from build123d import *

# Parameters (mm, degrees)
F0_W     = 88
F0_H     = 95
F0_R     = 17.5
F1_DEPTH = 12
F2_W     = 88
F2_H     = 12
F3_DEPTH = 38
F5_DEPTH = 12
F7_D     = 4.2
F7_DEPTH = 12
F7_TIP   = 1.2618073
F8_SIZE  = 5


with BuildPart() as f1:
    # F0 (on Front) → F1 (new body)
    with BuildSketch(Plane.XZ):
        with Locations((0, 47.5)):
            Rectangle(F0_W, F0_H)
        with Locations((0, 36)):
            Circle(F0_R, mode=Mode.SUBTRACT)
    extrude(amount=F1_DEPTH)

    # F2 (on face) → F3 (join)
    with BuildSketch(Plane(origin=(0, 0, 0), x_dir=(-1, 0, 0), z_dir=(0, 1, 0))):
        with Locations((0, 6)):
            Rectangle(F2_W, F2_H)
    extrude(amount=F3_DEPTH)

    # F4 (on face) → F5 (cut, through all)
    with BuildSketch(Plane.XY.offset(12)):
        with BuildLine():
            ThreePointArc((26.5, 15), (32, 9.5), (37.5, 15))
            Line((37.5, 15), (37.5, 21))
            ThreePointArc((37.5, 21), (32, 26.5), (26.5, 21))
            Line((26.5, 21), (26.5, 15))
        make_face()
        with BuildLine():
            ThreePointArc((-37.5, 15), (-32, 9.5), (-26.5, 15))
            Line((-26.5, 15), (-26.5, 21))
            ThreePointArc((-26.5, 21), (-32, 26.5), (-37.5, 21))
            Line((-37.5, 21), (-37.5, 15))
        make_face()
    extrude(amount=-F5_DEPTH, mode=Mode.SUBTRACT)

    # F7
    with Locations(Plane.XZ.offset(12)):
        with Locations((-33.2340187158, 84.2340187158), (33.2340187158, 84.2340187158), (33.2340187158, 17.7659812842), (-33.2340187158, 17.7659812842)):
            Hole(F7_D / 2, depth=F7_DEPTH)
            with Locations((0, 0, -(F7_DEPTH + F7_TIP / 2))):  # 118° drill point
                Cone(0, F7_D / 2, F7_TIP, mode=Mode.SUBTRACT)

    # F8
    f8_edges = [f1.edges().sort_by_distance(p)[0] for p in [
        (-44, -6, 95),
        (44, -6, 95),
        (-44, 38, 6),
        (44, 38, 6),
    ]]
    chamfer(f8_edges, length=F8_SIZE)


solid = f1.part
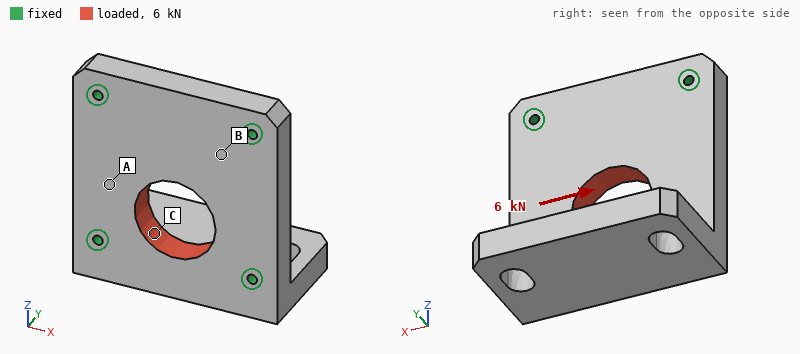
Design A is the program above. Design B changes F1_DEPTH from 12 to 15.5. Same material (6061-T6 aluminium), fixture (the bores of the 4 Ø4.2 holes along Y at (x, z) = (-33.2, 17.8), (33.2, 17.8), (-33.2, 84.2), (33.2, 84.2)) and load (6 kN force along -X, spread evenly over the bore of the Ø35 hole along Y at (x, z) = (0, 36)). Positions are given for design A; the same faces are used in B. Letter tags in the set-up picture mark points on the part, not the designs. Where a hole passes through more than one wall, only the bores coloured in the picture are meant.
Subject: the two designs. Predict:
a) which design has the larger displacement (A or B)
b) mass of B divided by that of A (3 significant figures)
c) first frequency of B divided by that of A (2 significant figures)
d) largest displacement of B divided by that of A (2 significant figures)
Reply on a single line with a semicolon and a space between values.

A; 1.21; 1.2; 0.77
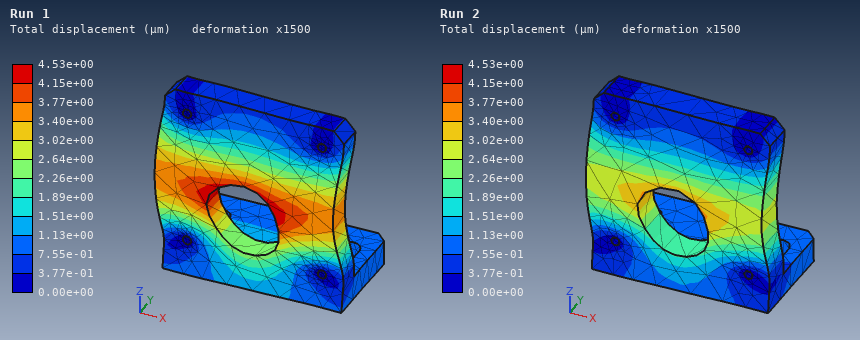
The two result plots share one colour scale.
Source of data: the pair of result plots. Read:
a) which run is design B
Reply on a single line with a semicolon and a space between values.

Run 2
